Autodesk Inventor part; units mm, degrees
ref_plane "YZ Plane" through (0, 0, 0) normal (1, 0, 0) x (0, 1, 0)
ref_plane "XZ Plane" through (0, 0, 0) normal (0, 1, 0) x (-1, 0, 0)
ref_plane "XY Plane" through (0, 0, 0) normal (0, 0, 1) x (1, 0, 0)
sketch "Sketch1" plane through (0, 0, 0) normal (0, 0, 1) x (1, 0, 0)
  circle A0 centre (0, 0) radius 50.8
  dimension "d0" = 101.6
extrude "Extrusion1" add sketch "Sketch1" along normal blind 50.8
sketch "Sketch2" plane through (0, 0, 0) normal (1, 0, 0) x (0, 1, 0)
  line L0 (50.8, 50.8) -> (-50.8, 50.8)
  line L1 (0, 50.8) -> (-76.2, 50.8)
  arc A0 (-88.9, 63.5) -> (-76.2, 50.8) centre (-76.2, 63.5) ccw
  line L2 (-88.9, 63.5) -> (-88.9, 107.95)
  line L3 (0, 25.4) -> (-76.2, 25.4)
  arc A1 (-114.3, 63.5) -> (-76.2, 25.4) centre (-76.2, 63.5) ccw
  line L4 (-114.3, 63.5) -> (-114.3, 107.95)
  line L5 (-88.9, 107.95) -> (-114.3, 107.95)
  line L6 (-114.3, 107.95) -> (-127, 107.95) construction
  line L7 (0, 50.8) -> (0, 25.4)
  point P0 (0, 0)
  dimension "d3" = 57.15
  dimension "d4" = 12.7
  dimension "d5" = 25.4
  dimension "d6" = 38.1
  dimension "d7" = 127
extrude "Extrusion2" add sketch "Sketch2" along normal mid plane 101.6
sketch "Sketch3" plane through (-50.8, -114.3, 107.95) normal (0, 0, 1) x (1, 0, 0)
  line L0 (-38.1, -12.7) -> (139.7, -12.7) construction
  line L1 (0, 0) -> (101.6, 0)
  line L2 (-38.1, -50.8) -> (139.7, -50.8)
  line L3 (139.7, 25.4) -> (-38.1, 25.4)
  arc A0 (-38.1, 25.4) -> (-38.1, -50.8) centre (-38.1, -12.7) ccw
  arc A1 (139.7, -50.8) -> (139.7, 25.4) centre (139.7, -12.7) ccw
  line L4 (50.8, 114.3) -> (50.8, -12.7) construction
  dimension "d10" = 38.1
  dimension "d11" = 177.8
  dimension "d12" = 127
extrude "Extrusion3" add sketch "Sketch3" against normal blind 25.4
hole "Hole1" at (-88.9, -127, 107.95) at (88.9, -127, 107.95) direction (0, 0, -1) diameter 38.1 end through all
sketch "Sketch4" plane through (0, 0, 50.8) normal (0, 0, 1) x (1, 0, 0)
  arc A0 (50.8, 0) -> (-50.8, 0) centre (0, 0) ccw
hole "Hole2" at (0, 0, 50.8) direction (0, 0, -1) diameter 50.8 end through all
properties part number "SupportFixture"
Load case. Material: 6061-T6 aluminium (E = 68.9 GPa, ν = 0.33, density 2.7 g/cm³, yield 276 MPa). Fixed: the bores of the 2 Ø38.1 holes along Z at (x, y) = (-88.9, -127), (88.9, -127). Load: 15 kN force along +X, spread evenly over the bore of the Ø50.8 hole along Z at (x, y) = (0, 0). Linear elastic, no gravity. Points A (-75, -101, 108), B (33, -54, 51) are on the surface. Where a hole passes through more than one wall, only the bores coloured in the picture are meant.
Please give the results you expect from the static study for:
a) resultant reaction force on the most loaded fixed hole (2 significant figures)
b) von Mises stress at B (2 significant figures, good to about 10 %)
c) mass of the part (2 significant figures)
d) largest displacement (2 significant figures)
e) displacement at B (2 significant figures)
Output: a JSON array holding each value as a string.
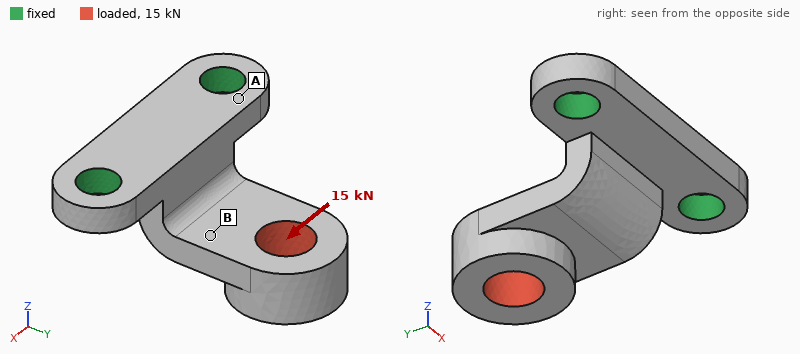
["17 kN", "22 MPa", "2.6 kg", "0.57 mm", "0.21 mm"]
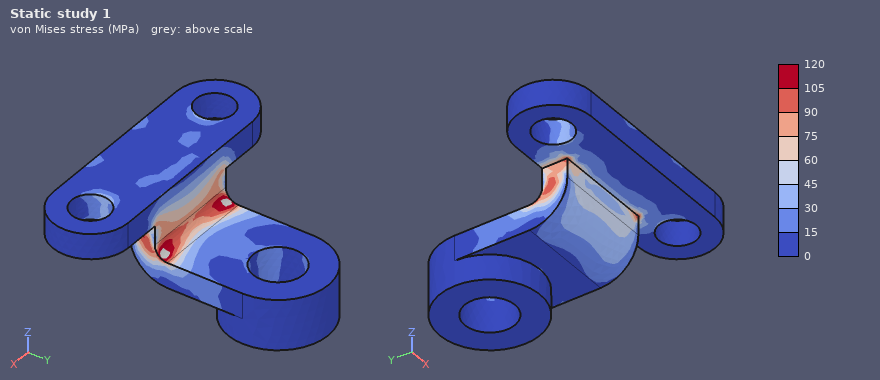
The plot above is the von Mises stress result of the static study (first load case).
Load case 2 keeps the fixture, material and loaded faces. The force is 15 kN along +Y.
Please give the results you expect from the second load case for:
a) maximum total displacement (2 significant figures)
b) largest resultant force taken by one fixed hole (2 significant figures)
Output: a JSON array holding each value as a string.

["1.2 mm", "7.5 kN"]
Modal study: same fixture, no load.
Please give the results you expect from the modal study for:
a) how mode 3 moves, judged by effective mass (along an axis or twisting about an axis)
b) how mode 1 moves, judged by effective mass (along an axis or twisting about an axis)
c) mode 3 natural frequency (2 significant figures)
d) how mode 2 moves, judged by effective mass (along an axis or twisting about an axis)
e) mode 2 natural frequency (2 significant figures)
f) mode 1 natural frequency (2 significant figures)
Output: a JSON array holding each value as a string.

["along Y", "along Z", "1900 Hz", "along X", "980 Hz", "440 Hz"]
